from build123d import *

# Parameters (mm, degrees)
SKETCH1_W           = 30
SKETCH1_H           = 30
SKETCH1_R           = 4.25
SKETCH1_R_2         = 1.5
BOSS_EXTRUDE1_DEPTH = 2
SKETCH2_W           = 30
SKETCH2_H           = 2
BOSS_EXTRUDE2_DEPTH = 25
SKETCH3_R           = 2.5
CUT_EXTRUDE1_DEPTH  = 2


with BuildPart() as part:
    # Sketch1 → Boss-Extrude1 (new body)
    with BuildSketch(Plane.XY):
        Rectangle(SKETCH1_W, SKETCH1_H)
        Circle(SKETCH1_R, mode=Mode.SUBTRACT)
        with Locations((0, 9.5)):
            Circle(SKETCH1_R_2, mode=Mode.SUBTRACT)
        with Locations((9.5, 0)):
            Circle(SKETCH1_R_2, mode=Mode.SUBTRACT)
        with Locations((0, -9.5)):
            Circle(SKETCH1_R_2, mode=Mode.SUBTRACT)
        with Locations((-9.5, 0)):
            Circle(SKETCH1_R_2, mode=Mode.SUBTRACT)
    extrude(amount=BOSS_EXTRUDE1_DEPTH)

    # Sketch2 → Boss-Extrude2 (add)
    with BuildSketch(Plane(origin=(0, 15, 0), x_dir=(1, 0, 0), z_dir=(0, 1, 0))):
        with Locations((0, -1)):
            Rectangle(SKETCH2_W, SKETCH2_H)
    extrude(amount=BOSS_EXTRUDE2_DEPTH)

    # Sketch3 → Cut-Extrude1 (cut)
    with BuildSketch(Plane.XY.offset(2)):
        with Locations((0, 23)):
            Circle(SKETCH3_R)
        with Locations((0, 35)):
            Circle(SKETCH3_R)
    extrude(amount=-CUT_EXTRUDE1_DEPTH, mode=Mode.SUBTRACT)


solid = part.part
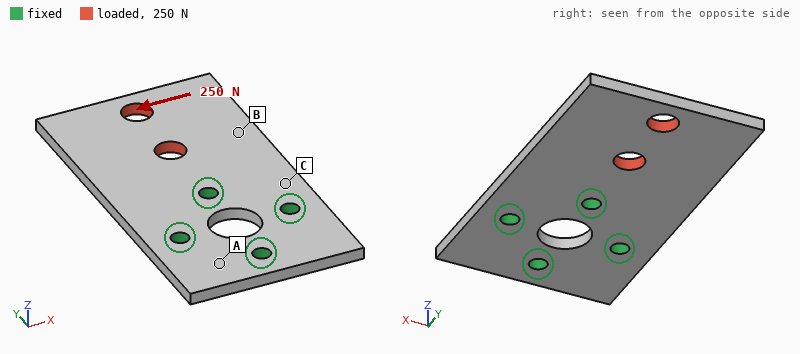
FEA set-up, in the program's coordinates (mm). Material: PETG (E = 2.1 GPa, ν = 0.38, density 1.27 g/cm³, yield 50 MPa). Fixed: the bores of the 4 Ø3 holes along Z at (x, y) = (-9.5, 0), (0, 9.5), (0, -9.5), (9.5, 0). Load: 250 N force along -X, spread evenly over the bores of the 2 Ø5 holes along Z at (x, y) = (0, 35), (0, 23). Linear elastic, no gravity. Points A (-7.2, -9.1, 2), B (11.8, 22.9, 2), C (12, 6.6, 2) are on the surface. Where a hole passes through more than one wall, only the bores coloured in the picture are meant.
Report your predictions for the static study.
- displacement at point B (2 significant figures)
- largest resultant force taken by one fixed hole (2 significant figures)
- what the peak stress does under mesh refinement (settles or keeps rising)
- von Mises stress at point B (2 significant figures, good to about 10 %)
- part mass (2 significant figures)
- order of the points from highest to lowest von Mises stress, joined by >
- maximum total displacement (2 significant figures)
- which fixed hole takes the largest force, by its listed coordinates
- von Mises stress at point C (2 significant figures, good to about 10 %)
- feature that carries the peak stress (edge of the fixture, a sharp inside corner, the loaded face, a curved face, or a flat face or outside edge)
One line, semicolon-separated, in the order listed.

0.24 mm; 290 N; keeps rising; 6.3 MPa; 3.9 g; C > B > A; 0.49 mm; (0, 9.5); 13 MPa; edge of the fixture
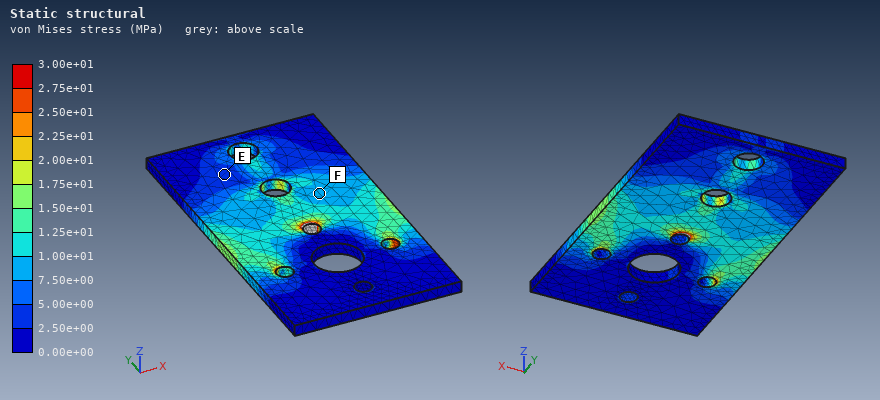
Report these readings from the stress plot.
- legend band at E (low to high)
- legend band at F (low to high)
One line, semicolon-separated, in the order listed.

2.50e+00 to 5.00e+00 MPa; 7.50e+00 to 1.00e+01 MPa
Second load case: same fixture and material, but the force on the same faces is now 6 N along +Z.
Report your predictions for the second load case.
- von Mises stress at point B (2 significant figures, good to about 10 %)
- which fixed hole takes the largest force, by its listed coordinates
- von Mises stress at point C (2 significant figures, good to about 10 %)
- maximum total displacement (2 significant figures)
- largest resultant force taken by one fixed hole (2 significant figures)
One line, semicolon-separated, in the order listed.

2.3 MPa; (0, 9.5); 1.7 MPa; 0.74 mm; 11 N
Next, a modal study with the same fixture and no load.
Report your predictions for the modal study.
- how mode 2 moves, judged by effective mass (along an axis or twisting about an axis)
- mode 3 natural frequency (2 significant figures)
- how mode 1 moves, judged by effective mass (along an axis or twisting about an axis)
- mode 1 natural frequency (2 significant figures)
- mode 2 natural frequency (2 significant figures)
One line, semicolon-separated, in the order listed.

twisting about Y; 2200 Hz; along Z; 440 Hz; 830 Hz
